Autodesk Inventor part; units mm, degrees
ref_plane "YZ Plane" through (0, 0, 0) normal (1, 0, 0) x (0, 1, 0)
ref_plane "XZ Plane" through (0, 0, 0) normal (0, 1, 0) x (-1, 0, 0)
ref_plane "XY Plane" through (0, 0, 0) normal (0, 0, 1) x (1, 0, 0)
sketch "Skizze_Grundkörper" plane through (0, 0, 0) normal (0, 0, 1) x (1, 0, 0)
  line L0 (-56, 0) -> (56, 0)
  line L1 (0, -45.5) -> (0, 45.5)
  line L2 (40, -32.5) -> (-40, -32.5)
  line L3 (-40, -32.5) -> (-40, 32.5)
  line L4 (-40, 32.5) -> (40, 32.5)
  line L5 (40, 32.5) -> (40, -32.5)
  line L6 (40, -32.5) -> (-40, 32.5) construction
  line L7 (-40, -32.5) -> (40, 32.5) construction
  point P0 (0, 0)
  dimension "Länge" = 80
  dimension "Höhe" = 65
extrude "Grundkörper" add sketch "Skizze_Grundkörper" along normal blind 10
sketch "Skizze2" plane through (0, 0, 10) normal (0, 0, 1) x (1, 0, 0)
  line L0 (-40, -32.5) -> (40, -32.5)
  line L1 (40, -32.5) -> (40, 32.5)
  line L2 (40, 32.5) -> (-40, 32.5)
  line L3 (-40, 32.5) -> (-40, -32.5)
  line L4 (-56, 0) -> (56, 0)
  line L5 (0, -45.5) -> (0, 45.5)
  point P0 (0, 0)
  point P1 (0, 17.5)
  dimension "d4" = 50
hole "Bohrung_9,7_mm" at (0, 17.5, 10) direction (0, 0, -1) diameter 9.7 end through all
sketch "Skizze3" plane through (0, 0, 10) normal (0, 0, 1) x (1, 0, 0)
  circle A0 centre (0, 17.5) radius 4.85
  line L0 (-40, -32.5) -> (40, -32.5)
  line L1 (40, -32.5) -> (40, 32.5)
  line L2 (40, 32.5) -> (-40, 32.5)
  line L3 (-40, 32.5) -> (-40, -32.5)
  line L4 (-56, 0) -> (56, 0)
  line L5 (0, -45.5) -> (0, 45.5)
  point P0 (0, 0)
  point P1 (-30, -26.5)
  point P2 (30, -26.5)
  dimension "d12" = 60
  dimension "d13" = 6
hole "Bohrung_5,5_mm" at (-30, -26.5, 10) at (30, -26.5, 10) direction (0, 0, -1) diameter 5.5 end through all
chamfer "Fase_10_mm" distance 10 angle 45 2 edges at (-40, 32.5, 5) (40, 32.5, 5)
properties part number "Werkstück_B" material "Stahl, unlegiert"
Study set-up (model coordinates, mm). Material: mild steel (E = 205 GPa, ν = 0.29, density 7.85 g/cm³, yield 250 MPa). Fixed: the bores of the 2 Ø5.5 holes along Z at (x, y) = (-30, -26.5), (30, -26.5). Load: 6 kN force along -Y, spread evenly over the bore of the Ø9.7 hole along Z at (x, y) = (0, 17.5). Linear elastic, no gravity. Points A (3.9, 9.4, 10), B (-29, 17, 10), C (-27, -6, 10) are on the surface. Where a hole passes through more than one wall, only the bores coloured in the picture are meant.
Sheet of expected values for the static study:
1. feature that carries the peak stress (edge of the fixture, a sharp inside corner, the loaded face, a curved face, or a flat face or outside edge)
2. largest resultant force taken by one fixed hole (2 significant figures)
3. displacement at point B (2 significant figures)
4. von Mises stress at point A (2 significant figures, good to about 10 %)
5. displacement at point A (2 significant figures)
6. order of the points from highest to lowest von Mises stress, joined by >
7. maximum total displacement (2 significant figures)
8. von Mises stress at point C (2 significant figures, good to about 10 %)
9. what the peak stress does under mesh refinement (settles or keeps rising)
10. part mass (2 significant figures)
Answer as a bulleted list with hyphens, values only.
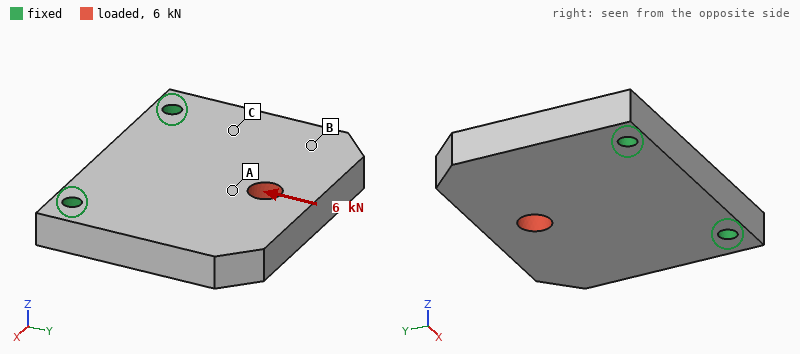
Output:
- edge of the fixture
- 3.2 kN
- 1.8 µm
- 18 MPa
- 3.5 µm
- A > C > B
- 5.1 µm
- 11 MPa
- keeps rising
- 390 g
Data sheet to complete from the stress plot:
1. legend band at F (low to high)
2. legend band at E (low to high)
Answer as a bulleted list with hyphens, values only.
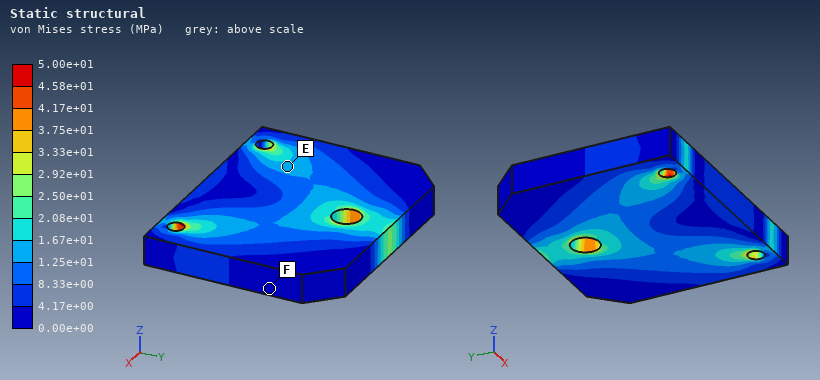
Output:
- 0.00e+00 to 4.17e+00 MPa
- 1.25e+01 to 1.67e+01 MPa
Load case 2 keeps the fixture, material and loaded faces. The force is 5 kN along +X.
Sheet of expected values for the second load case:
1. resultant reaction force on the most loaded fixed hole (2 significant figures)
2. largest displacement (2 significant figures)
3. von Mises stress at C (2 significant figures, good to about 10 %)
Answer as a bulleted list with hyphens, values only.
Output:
- 4.3 kN
- 8.3 µm
- 13 MPa
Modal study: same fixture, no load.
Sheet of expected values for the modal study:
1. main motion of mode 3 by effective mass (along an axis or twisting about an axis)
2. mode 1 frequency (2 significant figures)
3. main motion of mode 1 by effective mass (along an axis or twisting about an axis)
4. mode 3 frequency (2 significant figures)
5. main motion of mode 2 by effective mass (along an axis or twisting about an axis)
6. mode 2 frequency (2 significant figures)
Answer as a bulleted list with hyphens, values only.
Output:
- along X
- 2000 Hz
- along Z
- 9400 Hz
- twisting about Y
- 4600 Hz
